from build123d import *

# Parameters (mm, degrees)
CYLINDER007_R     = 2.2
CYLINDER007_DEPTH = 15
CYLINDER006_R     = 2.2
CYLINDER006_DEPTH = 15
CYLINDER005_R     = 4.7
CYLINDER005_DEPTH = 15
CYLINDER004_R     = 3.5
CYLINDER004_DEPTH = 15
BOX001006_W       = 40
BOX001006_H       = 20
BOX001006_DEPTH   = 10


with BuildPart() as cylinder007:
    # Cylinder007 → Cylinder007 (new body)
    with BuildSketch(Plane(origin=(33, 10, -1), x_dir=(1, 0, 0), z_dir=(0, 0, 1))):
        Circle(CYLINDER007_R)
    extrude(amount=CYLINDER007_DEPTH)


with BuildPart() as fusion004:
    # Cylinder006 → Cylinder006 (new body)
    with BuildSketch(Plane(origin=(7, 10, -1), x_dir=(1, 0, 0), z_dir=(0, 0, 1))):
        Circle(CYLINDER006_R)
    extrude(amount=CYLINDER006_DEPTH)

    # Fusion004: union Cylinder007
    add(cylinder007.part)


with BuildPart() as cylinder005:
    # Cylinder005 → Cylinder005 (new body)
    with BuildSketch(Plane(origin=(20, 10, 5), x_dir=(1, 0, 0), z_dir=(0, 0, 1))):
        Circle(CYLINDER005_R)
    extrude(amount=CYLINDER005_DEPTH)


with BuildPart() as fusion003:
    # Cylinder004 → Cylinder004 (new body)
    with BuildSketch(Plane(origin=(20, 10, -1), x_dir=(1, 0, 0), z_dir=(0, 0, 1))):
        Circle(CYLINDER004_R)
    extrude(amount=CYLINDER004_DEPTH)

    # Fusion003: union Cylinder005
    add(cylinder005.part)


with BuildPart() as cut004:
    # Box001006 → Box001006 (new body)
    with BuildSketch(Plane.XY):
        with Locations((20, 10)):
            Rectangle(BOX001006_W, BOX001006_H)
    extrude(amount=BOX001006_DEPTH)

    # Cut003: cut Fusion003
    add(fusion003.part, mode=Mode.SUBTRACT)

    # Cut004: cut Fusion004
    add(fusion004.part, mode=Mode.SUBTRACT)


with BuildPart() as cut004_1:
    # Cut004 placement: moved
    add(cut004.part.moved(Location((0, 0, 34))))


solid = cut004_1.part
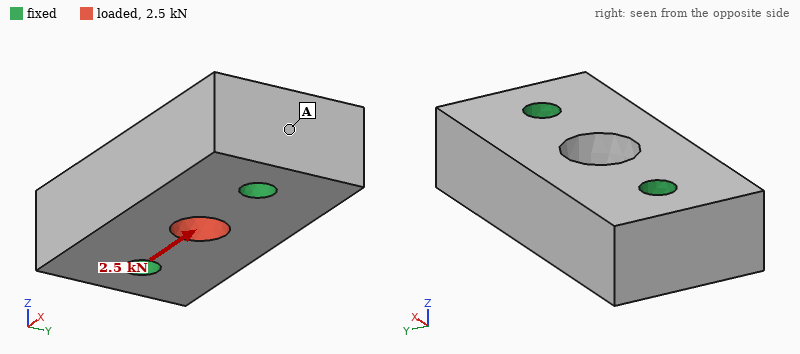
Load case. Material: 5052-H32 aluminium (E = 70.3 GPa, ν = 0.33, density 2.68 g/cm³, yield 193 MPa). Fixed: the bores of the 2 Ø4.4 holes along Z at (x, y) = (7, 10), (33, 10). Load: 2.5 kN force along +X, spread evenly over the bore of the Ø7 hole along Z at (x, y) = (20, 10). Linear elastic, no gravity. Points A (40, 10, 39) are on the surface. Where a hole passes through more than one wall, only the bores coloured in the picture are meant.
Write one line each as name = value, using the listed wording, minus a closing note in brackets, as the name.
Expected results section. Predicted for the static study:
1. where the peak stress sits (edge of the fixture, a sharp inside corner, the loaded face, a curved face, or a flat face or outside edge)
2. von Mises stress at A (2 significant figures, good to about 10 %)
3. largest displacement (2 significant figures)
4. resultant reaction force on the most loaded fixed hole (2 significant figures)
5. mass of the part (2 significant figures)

where the peak stress sits = a sharp inside corner
von Mises stress at A = 5.3 MPa
largest displacement = 2.9 µm
resultant reaction force on the most loaded fixed hole = 1.3 kN
mass of the part = 19 g
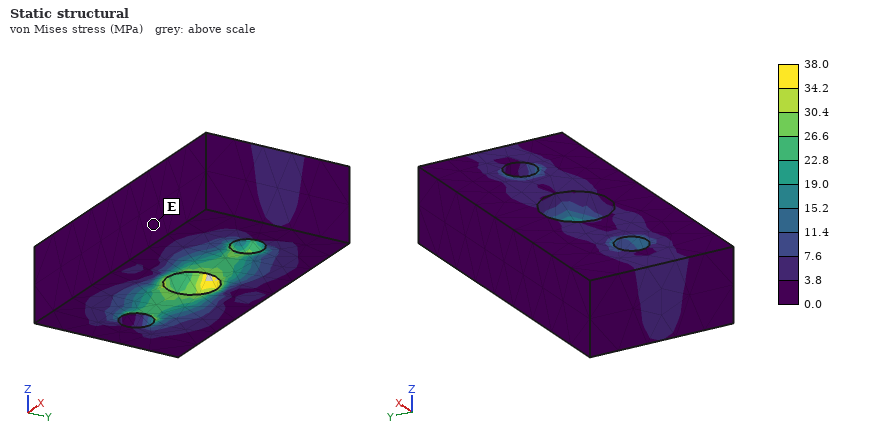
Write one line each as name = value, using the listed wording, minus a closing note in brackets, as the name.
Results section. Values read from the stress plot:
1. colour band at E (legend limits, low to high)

colour band at E = 0.0 to 3.8 MPa
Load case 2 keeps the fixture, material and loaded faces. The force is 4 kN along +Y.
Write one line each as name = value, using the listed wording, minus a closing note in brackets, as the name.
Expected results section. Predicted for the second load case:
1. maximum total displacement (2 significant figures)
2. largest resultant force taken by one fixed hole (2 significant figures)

maximum total displacement = 11 µm
largest resultant force taken by one fixed hole = 2.0 kN
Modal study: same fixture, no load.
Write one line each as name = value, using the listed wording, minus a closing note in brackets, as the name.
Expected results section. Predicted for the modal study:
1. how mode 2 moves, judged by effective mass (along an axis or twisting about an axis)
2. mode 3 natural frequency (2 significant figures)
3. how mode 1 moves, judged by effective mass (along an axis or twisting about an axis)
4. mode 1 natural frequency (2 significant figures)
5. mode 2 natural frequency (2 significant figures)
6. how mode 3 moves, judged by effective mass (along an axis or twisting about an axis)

how mode 2 moves, judged by effective mass = along Z
mode 3 natural frequency = 49 kHz
how mode 1 moves, judged by effective mass = twisting about X
mode 1 natural frequency = 39 kHz
mode 2 natural frequency = 42 kHz
how mode 3 moves, judged by effective mass = along Y
